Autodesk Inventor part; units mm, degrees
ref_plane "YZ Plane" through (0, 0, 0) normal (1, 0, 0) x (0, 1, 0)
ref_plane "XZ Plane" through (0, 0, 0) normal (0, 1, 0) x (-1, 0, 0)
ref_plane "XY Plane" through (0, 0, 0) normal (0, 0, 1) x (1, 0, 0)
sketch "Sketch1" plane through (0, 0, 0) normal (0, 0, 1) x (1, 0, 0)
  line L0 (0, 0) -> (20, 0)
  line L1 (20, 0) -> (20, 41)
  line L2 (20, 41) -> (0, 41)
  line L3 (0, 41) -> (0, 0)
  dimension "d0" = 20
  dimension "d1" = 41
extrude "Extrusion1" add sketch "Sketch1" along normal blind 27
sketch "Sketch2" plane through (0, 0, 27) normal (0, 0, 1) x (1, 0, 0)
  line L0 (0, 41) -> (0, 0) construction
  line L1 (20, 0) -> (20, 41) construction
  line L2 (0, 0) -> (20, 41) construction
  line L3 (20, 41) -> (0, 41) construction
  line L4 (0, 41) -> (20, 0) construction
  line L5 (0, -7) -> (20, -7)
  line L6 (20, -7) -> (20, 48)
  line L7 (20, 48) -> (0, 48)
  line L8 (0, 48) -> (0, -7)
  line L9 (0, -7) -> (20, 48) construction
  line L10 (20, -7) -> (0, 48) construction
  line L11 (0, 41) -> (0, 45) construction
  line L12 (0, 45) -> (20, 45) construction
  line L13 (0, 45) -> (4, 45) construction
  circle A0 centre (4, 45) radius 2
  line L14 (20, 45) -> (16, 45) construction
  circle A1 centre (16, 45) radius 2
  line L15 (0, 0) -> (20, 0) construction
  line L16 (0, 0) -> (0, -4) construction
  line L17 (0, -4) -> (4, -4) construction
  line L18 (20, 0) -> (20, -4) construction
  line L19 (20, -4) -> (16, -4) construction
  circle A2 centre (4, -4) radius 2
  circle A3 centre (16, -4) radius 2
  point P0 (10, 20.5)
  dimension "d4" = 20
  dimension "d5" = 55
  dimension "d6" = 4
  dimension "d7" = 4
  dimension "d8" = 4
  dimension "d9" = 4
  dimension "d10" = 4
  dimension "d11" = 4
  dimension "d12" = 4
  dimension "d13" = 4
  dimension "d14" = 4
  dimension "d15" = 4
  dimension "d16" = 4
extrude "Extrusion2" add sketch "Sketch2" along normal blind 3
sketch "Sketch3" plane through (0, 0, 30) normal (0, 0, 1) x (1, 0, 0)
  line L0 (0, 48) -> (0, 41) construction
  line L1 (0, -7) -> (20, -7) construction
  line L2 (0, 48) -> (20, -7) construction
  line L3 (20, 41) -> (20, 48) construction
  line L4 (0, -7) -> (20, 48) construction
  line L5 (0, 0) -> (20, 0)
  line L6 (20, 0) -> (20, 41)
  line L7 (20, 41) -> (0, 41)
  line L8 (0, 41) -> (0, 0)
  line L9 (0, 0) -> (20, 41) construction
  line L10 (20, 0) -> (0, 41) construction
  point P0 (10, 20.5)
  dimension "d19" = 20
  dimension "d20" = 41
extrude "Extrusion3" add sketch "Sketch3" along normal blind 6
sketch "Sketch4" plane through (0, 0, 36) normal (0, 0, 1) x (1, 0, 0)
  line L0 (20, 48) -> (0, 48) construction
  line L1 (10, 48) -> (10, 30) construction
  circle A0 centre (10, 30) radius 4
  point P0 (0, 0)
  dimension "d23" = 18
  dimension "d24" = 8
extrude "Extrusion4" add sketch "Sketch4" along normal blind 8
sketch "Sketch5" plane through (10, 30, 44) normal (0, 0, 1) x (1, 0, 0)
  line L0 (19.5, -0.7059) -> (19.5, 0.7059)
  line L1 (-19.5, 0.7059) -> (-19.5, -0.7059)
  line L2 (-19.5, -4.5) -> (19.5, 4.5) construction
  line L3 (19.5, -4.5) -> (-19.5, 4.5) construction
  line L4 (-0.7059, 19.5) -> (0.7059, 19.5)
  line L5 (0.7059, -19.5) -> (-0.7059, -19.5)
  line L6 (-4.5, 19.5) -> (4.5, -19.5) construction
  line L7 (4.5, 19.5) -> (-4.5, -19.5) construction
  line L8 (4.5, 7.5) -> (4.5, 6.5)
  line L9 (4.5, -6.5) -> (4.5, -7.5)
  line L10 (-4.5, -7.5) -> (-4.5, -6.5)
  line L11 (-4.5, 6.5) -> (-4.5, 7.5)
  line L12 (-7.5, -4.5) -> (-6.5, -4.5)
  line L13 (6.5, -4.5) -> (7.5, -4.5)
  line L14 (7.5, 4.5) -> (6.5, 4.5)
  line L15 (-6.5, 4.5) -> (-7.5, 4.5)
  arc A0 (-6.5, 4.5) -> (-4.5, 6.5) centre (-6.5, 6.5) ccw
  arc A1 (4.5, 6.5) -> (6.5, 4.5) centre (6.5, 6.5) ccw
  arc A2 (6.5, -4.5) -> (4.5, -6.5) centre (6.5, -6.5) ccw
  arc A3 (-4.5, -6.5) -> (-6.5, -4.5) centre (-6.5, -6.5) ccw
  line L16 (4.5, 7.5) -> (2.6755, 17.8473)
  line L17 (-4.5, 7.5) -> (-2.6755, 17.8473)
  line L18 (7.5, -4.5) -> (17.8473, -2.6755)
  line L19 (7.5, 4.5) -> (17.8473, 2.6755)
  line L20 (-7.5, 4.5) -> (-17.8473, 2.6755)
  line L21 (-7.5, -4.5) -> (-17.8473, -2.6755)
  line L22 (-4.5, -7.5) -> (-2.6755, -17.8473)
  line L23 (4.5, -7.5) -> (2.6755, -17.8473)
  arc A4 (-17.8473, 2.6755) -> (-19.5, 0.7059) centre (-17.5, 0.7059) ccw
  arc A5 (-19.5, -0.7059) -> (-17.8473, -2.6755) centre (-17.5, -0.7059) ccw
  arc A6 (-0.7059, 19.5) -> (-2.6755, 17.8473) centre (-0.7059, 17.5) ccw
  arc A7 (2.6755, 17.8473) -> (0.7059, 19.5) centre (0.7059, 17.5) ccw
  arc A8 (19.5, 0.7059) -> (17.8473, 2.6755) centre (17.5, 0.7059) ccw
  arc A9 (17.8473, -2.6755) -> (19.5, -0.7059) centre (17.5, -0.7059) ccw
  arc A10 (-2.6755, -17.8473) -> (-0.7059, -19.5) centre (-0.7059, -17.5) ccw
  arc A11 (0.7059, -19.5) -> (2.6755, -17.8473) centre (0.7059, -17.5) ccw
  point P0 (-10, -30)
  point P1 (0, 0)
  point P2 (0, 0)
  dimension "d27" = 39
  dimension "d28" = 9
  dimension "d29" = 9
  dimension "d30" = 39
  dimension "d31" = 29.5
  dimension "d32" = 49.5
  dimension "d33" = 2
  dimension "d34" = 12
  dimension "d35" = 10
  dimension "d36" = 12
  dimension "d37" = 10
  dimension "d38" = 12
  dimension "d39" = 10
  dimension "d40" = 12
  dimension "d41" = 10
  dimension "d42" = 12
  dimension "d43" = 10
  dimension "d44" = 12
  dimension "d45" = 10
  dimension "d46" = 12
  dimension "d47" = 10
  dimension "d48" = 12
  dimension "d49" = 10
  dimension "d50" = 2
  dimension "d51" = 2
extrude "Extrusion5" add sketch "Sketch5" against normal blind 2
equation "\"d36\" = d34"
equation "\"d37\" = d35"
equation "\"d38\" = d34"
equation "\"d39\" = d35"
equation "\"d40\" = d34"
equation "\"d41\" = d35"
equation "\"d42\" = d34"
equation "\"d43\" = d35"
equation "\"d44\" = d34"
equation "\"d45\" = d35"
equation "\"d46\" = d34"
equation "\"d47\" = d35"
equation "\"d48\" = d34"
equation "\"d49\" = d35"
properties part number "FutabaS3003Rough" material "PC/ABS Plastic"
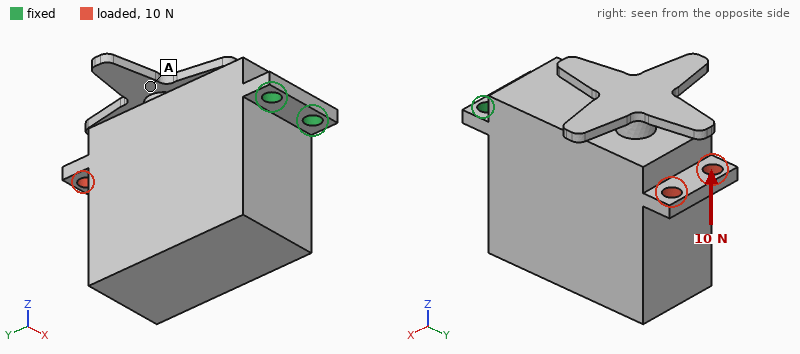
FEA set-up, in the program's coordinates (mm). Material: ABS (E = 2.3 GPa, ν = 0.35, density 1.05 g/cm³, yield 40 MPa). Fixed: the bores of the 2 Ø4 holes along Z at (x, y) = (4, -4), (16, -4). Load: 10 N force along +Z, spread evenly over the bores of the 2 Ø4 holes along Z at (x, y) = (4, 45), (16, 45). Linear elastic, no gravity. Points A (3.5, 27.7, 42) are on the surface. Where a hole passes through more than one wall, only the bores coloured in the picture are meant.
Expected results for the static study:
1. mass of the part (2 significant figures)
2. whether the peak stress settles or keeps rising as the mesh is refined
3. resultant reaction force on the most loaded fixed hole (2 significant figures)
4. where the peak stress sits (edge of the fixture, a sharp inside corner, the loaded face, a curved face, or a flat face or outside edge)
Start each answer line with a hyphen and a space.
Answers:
- 33 g
- keeps rising
- 5.0 N
- edge of the fixture
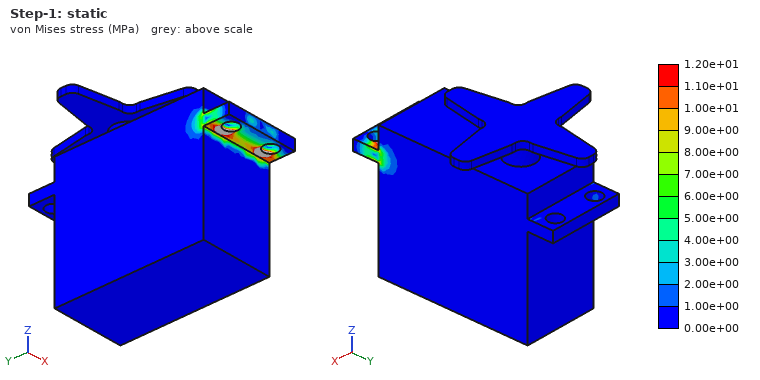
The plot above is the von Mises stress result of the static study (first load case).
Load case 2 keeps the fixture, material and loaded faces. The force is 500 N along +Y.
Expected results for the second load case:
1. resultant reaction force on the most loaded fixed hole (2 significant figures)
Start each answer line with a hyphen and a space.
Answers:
- 250 N
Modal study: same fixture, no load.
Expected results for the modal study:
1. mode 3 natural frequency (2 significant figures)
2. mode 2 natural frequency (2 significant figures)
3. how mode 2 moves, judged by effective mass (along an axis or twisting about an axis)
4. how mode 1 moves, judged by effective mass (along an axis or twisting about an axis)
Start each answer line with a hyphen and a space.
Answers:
- 1100 Hz
- 710 Hz
- along X
- along Z
